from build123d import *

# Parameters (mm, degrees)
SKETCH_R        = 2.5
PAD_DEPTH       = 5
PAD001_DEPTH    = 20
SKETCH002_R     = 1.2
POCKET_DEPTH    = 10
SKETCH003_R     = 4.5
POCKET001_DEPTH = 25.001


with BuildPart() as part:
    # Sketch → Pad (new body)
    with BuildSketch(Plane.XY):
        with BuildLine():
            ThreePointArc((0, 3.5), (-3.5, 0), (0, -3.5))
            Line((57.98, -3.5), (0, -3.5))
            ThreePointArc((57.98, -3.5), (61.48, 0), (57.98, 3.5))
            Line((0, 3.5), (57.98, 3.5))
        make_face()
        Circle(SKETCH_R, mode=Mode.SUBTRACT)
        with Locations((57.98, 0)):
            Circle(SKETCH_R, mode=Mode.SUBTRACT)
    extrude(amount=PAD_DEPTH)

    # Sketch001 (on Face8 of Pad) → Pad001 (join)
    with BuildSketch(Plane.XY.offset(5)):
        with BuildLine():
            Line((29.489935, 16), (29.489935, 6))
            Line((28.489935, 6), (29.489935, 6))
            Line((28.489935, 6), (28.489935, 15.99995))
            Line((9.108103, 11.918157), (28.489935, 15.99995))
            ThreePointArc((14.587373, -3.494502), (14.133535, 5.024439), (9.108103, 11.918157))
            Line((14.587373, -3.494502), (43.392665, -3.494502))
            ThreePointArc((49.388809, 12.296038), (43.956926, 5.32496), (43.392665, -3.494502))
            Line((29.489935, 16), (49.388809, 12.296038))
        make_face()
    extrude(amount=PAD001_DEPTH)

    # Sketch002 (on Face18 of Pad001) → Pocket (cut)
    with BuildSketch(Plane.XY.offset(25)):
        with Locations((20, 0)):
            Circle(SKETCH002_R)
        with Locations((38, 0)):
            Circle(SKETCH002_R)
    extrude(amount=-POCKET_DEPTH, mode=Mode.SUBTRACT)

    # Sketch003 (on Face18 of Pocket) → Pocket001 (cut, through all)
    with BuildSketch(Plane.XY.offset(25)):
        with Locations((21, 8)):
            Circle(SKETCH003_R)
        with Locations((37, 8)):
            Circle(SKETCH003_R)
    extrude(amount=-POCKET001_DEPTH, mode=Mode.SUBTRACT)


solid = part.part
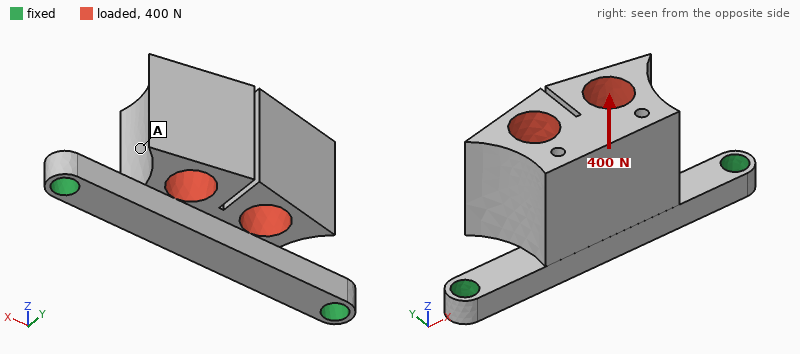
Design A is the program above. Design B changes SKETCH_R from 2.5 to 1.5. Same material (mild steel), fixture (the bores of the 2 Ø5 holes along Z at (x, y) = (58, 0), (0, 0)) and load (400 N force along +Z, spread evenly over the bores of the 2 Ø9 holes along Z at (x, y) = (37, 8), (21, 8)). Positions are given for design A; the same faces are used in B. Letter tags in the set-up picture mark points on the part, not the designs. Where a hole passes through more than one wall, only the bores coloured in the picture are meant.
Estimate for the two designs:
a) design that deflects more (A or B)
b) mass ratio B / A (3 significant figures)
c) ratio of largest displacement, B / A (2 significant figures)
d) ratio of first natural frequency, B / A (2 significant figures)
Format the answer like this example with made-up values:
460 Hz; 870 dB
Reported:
B; 1.01; 1.1; 0.95
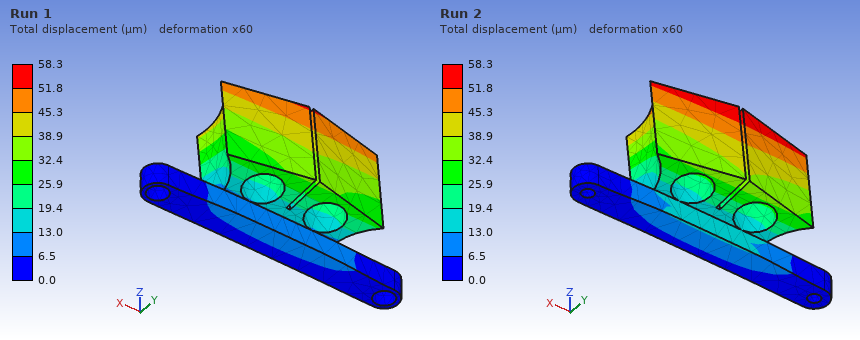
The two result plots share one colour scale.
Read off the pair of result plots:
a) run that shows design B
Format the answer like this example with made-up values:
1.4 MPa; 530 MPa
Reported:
Run 2
